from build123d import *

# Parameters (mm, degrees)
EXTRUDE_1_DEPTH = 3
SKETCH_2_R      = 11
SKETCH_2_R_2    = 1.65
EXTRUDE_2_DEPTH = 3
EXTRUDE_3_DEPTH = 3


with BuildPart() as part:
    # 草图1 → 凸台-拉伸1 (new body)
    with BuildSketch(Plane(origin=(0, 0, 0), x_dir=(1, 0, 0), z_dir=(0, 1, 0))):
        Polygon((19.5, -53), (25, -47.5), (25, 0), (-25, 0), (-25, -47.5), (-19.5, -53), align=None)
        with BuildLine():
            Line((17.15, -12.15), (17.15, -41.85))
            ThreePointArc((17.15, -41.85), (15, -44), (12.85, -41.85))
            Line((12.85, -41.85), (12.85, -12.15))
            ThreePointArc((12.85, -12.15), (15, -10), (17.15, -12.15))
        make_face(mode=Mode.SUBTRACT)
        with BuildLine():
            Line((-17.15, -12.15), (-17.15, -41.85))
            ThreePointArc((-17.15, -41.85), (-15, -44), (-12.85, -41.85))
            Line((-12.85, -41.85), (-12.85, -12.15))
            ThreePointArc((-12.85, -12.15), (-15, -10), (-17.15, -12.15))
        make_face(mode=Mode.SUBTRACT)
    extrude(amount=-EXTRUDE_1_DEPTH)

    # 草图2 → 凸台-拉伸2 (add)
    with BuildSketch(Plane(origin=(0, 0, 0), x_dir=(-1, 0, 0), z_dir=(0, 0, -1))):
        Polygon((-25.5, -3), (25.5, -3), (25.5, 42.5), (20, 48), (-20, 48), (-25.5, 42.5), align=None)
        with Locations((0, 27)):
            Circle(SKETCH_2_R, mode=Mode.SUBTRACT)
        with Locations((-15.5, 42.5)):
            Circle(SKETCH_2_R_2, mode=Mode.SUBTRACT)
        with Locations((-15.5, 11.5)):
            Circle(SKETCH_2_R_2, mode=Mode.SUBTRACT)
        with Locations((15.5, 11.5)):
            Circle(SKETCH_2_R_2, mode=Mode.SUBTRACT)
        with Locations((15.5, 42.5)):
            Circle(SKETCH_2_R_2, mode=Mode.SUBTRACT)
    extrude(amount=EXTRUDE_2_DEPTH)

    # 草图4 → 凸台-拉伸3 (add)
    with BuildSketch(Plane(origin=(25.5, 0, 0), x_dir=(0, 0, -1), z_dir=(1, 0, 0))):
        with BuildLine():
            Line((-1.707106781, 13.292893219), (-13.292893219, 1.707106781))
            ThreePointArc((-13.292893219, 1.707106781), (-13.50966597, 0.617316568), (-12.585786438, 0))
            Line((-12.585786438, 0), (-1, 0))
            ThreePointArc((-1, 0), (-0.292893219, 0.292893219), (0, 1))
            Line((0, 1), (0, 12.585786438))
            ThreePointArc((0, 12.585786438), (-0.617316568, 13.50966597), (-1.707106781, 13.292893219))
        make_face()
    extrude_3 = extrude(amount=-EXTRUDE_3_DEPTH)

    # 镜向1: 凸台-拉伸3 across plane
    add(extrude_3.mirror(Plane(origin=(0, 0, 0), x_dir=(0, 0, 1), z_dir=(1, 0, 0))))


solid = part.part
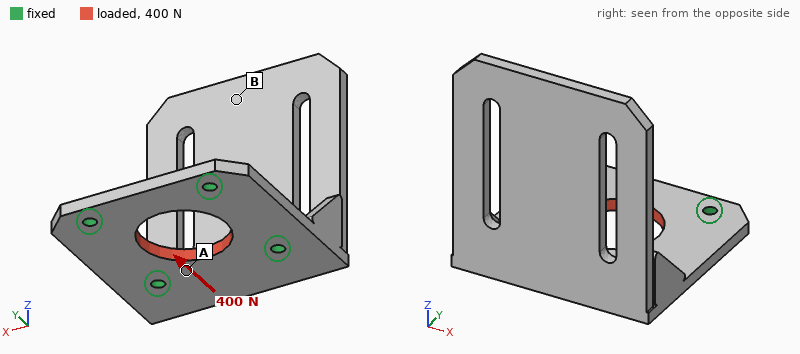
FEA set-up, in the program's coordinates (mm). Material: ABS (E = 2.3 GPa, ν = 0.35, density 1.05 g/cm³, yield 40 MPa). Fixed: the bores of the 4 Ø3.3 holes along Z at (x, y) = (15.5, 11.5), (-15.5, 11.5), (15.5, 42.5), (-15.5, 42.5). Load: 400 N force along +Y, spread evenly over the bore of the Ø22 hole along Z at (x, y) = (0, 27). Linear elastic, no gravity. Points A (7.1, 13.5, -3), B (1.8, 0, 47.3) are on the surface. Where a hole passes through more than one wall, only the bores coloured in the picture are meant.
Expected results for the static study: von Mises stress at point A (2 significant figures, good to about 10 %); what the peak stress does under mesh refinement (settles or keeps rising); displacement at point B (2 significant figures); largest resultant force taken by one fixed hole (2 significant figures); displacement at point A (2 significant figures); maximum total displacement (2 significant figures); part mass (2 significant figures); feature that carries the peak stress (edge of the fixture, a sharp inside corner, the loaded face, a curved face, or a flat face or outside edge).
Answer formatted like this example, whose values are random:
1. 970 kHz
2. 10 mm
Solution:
1. 1.6 MPa
2. keeps rising
3. 13 µm
4. 100 N
5. 14 µm
6. 38 µm
7. 15 g
8. edge of the fixture
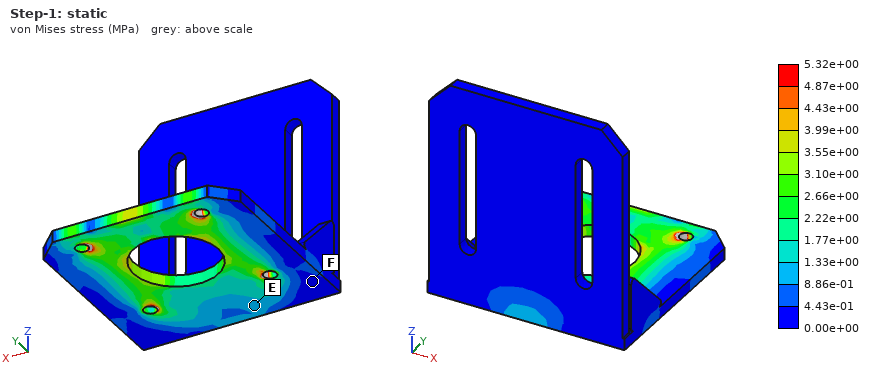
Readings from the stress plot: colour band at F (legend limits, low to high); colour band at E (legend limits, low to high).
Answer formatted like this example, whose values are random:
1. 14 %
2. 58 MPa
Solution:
1. 0.00e+00 to 4.43e-01 MPa
2. 8.86e-01 to 1.33e+00 MPa
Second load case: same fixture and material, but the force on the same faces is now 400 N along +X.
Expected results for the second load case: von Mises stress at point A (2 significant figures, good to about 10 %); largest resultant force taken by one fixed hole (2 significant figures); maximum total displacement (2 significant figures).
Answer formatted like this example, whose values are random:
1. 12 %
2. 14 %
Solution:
1. 2.6 MPa
2. 100 N
3. 28 µm
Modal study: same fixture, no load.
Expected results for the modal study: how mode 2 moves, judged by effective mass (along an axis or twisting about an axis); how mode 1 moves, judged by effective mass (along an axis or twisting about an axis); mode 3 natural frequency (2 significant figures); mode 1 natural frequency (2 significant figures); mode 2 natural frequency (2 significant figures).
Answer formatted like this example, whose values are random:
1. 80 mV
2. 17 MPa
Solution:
1. along X
2. along Y
3. 870 Hz
4. 230 Hz
5. 550 Hz
